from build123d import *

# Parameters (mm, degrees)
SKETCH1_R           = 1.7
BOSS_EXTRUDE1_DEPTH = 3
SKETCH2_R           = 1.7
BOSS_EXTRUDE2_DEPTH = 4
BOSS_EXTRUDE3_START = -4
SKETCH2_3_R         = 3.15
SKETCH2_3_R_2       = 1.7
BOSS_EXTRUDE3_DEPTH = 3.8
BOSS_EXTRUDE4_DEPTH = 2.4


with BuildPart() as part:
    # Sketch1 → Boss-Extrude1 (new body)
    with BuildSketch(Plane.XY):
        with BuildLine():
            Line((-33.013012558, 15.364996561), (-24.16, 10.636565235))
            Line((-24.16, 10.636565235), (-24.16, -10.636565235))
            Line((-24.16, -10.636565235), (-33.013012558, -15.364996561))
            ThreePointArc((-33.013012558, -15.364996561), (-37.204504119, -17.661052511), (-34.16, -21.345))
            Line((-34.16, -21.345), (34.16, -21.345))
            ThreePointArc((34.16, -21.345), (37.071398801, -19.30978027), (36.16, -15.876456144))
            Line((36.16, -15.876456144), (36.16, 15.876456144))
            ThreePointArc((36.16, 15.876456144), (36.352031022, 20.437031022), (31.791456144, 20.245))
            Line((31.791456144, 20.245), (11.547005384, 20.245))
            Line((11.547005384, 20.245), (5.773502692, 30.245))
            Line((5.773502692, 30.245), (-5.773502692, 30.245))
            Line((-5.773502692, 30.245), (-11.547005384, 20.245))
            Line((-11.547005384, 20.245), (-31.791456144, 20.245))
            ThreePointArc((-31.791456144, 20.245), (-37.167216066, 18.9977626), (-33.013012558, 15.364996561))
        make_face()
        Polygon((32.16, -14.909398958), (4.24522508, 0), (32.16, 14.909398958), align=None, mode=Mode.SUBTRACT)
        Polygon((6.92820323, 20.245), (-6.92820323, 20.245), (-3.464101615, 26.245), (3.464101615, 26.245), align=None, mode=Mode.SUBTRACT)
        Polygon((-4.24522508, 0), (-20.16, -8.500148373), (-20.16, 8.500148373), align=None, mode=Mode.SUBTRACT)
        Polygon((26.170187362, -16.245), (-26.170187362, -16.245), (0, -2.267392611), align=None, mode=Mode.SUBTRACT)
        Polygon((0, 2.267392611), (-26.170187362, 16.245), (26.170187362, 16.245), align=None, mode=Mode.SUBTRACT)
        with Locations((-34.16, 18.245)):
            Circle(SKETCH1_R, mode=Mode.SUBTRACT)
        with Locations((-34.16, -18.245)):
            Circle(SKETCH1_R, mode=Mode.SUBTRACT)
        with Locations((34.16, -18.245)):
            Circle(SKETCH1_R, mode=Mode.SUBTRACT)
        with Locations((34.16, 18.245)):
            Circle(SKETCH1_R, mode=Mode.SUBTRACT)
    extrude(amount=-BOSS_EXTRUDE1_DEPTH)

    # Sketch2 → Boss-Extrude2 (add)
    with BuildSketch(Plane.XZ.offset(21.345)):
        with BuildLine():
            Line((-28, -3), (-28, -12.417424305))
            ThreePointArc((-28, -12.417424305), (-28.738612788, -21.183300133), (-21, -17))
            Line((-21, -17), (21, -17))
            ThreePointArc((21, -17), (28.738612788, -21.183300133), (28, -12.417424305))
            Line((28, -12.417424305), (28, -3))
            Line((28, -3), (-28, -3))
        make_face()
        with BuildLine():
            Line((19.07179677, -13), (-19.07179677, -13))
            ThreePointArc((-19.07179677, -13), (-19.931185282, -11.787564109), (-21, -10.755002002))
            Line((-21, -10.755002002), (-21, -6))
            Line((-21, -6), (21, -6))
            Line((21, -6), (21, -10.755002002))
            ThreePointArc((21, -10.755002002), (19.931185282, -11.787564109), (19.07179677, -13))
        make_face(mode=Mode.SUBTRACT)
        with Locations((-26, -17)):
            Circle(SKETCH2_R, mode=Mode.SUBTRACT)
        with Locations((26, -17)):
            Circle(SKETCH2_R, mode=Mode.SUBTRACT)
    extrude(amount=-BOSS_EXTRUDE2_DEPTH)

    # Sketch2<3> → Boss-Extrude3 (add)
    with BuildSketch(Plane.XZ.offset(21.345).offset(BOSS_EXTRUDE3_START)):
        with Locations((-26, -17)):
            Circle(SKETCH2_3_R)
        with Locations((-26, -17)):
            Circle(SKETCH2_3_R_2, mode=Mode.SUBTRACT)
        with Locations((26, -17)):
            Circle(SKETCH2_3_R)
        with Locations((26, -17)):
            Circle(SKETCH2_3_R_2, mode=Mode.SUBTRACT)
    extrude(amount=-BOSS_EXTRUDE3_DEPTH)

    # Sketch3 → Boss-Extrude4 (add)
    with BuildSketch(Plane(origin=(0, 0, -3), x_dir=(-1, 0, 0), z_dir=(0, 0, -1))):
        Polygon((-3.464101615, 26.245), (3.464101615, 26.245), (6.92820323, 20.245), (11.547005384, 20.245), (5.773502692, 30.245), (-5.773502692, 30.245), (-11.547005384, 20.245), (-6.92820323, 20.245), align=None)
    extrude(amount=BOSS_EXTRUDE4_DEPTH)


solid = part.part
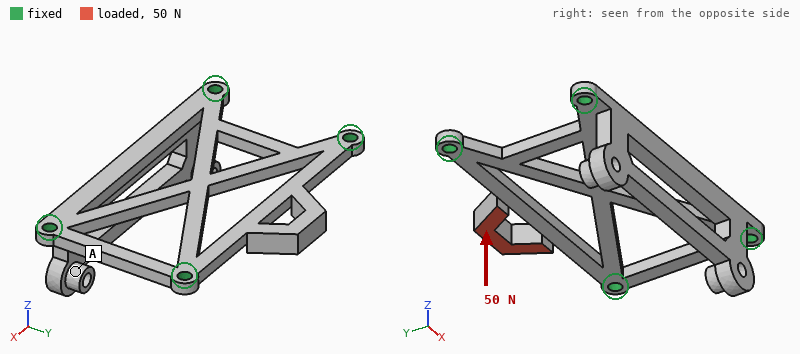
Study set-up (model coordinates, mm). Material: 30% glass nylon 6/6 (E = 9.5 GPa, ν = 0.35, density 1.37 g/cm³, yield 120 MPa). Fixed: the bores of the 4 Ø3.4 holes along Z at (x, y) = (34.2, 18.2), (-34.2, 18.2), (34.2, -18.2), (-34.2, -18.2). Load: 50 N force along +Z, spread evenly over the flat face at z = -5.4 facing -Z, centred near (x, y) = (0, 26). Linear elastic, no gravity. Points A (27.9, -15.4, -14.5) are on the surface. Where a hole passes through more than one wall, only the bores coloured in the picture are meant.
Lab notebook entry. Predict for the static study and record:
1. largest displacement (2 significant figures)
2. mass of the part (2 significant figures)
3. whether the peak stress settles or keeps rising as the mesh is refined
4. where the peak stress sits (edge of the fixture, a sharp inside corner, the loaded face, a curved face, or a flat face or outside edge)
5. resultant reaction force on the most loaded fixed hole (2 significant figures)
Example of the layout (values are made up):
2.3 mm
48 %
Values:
1.1 mm
9.9 g
keeps rising
edge of the fixture
26 N
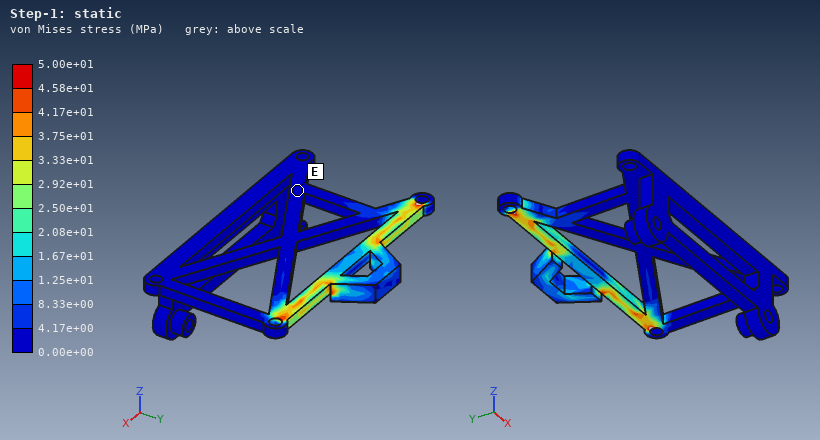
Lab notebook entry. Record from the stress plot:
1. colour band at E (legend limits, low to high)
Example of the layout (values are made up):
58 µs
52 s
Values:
0.00e+00 to 4.17e+00 MPa
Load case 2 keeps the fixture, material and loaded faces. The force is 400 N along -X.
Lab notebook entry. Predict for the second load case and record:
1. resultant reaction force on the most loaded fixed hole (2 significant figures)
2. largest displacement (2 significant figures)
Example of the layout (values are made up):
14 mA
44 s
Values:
200 N
0.36 mm
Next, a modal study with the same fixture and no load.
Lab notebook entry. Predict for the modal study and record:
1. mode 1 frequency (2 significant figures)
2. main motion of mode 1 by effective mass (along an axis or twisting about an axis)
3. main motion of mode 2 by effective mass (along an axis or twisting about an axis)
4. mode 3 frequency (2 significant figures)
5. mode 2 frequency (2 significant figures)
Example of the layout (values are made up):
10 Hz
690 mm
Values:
1200 Hz
along Z
along Y
1800 Hz
1400 Hz
